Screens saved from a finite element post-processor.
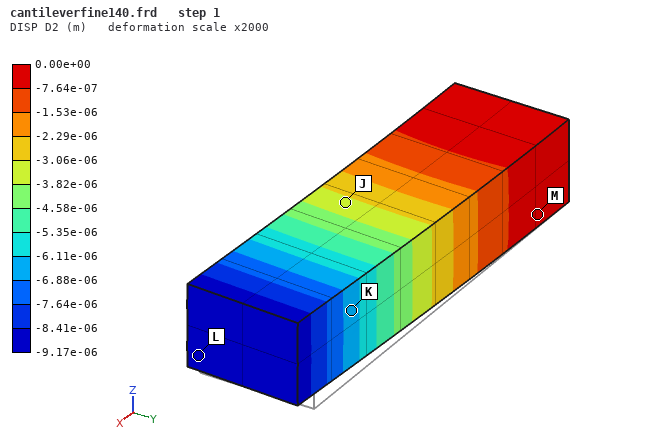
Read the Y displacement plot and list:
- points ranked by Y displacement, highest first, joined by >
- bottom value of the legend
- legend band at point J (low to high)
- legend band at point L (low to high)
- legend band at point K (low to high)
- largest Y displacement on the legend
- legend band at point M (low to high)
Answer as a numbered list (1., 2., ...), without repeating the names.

1. M > J > K > L
2. -9.17e-06 m
3. -3.82e-06 to -3.06e-06 m
4. -9.17e-06 to -8.41e-06 m
5. -6.88e-06 to -6.11e-06 m
6. 0.00e+00 m
7. -7.64e-07 to 0.00e+00 m
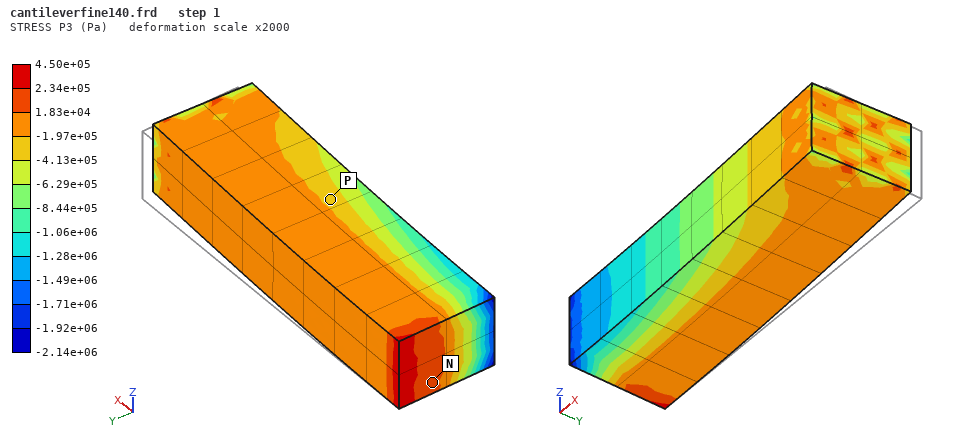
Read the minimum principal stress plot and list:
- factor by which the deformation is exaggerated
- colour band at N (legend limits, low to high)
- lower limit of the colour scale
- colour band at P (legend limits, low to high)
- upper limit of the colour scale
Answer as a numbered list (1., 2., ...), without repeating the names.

1. 2000
2. 1.83e+04 to 2.34e+05 Pa
3. -2.14e+06 Pa
4. -4.13e+05 to -1.97e+05 Pa
5. 4.50e+05 Pa
